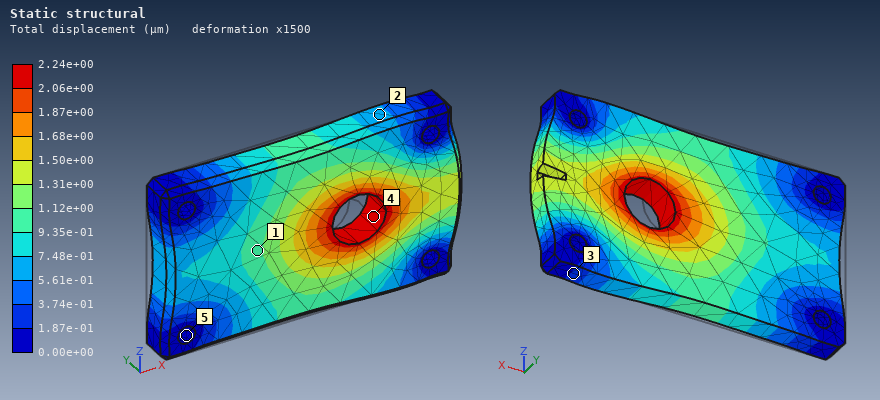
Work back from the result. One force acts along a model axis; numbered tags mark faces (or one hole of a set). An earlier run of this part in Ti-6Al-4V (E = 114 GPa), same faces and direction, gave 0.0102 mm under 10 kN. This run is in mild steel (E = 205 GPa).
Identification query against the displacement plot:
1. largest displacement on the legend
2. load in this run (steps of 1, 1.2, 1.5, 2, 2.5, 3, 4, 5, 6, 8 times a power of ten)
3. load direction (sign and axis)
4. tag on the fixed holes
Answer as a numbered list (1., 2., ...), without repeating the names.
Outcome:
1. 2.24e+00 µm
2. 4 kN
3. +X
4. 5
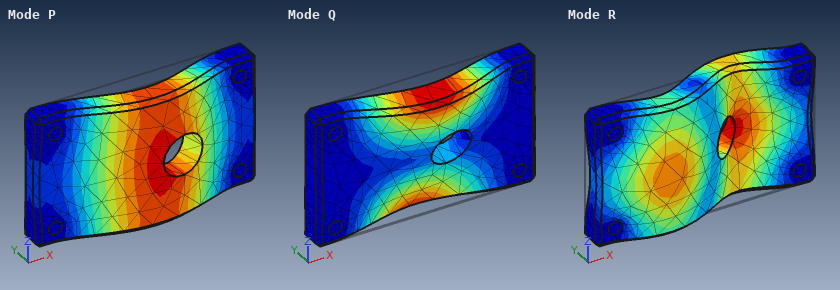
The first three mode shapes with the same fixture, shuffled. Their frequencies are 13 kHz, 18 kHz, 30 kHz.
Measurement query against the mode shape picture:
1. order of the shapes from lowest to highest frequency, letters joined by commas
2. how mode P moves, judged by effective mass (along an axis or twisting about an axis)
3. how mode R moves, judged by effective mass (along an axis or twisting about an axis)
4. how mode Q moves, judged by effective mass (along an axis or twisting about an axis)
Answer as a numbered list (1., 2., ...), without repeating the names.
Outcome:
1. P, Q, R
2. along Y
3. twisting about Z
4. twisting about X
